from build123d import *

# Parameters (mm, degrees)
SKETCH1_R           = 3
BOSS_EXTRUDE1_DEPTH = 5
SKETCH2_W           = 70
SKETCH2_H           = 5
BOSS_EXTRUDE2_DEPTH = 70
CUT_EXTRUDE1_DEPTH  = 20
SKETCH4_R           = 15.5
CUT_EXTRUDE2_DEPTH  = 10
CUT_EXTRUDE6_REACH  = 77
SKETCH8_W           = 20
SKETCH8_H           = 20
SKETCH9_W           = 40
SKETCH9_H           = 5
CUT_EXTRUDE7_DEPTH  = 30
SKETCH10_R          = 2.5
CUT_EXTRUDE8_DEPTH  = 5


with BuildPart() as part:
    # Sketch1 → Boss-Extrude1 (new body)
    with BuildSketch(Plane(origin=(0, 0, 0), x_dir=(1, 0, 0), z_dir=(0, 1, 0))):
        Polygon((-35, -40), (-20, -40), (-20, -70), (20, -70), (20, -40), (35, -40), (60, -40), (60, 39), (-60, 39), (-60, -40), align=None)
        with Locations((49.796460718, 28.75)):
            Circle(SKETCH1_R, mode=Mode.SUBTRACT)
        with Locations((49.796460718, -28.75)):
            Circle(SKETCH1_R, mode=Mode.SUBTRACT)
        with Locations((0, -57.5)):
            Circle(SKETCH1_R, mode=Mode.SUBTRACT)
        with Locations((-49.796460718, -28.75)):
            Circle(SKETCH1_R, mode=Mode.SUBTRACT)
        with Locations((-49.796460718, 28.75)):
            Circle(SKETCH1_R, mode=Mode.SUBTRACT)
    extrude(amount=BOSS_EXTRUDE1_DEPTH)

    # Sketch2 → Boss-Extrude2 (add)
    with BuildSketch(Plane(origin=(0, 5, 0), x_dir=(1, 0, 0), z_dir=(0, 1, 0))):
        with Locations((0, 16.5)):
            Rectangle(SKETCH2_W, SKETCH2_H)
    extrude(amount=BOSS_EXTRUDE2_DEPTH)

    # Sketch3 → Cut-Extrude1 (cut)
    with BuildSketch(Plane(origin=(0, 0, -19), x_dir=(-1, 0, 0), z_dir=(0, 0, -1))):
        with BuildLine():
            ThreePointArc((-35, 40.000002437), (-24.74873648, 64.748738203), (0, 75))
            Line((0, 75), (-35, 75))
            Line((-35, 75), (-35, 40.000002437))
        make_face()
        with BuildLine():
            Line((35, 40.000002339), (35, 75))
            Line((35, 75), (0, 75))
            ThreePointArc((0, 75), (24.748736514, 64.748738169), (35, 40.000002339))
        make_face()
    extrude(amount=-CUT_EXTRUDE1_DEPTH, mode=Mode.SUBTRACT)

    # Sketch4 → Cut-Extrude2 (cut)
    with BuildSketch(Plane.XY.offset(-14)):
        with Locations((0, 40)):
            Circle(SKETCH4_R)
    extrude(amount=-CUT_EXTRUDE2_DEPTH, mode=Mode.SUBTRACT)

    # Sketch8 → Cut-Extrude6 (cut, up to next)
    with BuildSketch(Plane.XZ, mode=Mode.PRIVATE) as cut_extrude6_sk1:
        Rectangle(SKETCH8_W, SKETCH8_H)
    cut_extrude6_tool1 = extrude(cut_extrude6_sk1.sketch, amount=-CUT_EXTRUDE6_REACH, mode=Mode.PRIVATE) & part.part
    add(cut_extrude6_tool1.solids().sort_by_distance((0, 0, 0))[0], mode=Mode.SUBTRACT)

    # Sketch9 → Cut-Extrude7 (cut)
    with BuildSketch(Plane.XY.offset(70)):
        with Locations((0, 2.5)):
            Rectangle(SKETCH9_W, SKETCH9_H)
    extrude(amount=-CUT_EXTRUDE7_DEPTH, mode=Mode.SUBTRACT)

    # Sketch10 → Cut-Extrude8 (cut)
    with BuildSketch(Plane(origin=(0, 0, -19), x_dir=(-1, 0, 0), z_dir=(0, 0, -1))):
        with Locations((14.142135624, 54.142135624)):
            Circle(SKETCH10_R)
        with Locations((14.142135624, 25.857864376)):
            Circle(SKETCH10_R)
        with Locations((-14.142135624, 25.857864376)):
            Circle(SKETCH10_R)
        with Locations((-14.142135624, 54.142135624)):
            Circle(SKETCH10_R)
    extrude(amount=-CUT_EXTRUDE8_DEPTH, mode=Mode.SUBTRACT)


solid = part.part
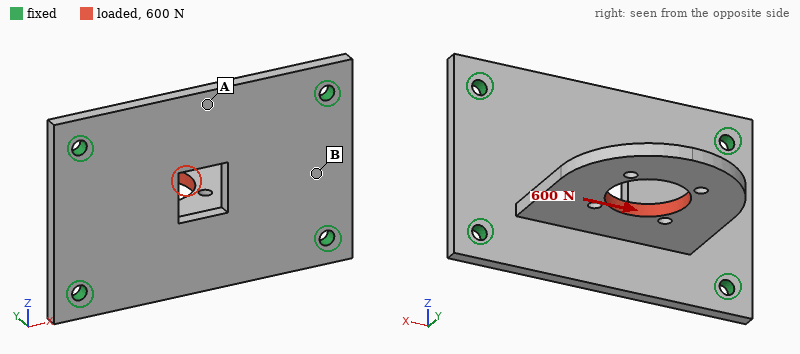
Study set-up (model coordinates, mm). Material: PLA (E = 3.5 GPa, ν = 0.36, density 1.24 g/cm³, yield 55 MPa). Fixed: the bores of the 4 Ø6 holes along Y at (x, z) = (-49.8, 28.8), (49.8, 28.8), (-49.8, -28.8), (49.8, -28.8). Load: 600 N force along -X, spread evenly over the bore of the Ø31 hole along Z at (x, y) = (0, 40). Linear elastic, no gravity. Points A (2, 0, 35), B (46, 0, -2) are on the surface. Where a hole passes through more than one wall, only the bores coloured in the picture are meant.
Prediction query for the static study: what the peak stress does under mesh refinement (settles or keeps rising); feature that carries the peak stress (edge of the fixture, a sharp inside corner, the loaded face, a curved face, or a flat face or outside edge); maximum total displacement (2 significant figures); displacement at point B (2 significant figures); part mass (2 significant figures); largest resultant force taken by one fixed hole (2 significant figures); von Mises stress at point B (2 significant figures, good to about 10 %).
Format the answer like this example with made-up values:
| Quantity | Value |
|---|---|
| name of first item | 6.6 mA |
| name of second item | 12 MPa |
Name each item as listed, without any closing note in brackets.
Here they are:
| Quantity | Value |
|---|---|
| what the peak stress does under mesh refinement | keeps rising |
| feature that carries the peak stress | edge of the fixture |
| maximum total displacement | 0.63 mm |
| displacement at point B | 0.11 mm |
| part mass | 78 g |
| largest resultant force taken by one fixed hole | 330 N |
| von Mises stress at point B | 4.6 MPa |
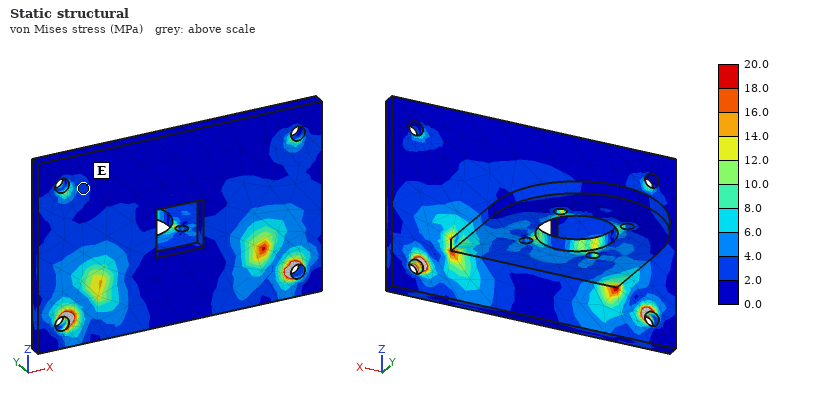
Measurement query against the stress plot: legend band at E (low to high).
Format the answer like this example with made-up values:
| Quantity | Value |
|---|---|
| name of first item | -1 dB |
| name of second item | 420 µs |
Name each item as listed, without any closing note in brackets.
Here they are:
| Quantity | Value |
|---|---|
| legend band at E | 2.0 to 4.0 MPa |
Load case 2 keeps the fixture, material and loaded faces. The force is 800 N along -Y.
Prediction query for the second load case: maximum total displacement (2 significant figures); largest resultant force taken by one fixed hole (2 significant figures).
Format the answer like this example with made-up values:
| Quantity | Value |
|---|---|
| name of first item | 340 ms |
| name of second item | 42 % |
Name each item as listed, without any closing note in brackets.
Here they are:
| Quantity | Value |
|---|---|
| maximum total displacement | 0.56 mm |
| largest resultant force taken by one fixed hole | 360 N |
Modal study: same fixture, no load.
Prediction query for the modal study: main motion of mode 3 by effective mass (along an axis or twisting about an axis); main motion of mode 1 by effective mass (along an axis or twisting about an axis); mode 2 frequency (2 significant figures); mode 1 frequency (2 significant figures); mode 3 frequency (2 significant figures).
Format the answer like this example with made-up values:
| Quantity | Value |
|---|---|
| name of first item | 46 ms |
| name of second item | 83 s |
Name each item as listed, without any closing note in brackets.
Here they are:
| Quantity | Value |
|---|---|
| main motion of mode 3 by effective mass | along Y |
| main motion of mode 1 by effective mass | along Z |
| mode 2 frequency | 740 Hz |
| mode 1 frequency | 270 Hz |
| mode 3 frequency | 940 Hz |
